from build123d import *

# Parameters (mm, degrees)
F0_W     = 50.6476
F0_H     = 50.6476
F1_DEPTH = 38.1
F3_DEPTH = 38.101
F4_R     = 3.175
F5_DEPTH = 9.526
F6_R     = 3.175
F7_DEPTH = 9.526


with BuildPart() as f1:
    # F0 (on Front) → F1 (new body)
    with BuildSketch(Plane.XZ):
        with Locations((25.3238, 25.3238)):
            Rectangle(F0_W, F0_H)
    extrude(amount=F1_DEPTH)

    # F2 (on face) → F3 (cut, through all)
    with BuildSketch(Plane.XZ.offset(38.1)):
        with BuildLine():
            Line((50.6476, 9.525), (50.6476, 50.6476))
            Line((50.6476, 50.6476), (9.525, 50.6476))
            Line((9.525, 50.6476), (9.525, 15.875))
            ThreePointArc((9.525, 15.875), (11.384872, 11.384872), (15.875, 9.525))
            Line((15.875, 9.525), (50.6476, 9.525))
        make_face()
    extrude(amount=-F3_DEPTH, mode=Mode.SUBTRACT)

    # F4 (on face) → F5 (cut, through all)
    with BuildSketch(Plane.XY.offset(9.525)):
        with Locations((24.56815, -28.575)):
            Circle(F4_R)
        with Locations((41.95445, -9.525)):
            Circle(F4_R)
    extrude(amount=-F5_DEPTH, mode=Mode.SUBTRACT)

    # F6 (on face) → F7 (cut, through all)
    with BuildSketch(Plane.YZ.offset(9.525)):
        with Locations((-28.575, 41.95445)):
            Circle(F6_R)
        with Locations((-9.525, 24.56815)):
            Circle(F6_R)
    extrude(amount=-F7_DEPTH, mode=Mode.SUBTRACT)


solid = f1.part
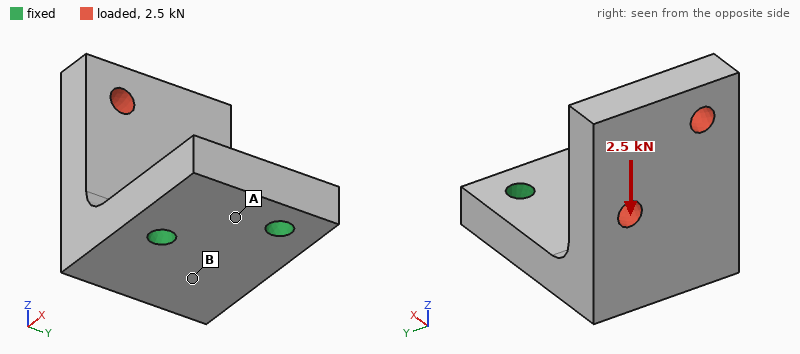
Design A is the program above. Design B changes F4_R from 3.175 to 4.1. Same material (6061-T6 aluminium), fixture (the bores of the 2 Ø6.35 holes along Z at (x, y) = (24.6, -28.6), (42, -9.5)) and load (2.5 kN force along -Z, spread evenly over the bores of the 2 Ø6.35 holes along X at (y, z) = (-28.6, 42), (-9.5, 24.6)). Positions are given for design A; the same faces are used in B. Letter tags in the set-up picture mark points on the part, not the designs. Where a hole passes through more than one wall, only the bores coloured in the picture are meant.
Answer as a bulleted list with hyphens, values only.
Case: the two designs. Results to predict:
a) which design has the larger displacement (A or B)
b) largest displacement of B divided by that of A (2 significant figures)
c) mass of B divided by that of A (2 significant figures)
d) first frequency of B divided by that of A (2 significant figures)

- A
- 0.88
- 0.99
- 1.0
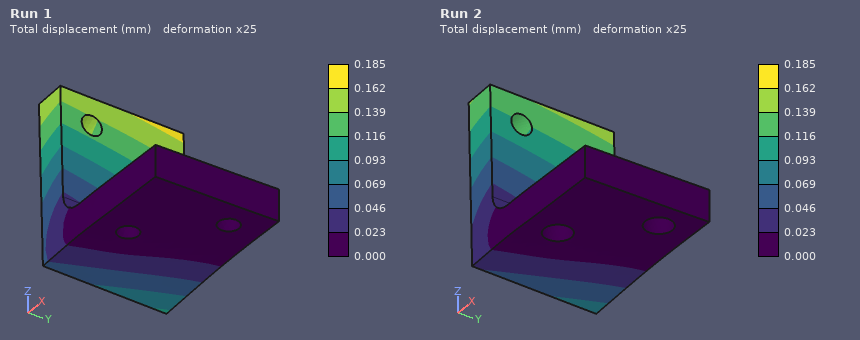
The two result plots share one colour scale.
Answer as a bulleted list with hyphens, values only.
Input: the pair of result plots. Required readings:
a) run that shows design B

- Run 2
